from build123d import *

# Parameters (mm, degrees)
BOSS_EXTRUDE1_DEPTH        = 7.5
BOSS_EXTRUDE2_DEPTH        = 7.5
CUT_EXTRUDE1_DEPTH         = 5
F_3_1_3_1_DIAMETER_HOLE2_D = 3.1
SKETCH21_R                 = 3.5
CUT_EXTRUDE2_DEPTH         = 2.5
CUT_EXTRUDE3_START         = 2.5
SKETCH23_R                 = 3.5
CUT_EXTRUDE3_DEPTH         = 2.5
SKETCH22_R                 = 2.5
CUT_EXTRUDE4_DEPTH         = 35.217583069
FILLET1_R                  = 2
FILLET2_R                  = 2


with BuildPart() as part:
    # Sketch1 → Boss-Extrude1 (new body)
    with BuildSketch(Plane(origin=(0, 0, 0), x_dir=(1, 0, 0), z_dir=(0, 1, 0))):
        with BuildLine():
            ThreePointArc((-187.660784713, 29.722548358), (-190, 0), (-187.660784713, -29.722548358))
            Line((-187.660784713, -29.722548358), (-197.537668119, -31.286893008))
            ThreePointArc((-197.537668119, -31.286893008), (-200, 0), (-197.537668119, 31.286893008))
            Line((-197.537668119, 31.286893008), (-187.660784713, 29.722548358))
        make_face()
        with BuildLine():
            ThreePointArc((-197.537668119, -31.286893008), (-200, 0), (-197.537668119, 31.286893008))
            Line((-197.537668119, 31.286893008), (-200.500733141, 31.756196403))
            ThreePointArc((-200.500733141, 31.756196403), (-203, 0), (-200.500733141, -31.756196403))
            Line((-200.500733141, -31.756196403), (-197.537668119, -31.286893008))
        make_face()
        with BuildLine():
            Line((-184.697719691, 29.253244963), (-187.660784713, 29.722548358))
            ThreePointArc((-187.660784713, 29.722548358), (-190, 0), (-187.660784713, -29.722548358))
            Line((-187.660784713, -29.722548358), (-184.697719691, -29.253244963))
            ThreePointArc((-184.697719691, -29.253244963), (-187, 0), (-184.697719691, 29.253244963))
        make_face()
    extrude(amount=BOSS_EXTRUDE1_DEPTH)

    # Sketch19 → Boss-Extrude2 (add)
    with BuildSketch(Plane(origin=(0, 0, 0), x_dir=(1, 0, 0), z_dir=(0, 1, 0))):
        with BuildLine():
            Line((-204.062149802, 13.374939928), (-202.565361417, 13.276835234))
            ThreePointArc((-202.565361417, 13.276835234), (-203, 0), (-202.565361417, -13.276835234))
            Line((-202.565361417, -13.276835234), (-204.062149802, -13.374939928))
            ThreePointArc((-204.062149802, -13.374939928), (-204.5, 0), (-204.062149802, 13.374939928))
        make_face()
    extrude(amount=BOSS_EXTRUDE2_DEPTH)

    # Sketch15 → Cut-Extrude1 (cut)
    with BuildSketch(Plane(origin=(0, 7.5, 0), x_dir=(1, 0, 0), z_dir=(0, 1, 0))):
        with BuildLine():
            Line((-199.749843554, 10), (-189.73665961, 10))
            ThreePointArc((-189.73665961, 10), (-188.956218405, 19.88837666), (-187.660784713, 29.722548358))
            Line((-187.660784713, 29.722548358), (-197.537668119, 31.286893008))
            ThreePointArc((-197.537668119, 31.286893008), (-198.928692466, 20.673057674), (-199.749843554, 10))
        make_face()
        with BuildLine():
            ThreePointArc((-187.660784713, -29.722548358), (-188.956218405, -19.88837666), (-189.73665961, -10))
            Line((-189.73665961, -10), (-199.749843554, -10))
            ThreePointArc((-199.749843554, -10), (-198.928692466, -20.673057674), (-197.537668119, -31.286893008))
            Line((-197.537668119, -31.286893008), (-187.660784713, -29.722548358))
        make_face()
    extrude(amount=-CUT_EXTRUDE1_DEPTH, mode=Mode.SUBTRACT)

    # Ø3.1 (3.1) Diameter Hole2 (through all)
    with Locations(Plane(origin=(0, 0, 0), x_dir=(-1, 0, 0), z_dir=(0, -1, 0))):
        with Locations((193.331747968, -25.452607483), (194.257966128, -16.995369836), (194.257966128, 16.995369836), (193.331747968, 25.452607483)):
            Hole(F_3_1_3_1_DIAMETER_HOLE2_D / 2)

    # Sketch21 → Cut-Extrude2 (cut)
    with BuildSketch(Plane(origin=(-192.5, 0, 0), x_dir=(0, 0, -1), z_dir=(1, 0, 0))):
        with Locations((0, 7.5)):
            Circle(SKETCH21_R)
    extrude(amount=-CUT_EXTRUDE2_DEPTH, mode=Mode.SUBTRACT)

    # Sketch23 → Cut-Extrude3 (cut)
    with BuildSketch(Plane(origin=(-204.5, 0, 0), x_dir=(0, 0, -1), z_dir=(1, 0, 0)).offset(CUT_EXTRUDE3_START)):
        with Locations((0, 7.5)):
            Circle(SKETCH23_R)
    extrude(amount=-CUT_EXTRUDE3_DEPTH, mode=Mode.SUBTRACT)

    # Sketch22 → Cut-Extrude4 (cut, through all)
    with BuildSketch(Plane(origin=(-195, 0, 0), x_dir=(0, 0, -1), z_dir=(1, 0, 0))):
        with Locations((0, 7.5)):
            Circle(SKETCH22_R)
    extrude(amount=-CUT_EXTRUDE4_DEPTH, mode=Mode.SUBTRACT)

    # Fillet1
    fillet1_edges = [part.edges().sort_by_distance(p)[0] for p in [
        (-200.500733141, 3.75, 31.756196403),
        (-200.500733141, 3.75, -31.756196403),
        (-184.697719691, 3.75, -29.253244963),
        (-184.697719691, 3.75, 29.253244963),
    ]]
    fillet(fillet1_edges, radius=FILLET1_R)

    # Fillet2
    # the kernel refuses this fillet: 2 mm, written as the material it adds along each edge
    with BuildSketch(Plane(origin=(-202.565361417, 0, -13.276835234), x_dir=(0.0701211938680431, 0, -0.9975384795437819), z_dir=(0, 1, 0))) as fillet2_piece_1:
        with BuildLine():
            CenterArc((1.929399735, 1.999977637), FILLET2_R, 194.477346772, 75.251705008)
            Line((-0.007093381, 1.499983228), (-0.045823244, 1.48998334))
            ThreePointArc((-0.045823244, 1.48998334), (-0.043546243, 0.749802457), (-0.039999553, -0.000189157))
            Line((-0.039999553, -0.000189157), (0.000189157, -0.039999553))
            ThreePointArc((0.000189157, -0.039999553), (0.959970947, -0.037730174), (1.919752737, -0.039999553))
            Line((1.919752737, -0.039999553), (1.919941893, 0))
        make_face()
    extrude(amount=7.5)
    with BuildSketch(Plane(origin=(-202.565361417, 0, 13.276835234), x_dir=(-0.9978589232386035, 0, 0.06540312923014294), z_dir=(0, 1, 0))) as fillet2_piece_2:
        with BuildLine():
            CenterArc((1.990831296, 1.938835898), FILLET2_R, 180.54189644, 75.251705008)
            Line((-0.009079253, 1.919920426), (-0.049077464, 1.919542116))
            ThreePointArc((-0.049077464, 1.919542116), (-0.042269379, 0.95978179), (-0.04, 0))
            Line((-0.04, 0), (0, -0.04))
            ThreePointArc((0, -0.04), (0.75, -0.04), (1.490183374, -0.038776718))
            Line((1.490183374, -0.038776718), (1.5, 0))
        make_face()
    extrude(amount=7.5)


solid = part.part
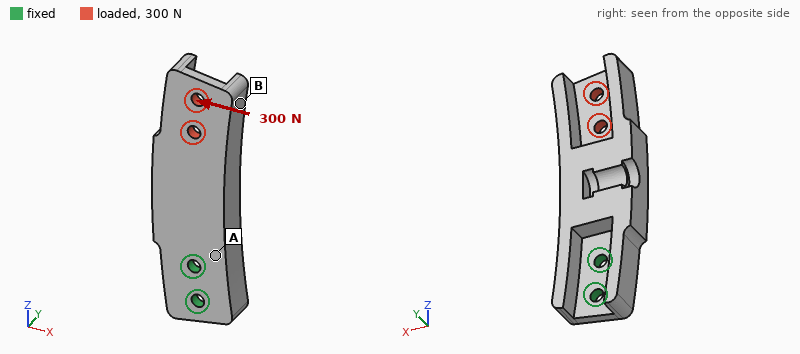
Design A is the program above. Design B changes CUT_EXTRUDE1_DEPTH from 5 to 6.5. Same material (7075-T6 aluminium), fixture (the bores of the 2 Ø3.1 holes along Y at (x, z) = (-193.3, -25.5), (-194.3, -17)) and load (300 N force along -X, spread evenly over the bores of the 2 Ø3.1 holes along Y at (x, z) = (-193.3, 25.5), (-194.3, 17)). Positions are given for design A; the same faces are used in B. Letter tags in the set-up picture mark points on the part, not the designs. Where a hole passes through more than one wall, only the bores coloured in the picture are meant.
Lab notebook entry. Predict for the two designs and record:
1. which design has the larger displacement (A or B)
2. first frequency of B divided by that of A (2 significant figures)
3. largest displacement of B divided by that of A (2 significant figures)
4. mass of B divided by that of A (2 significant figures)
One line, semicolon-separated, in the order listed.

B; 0.59; 2.0; 0.89
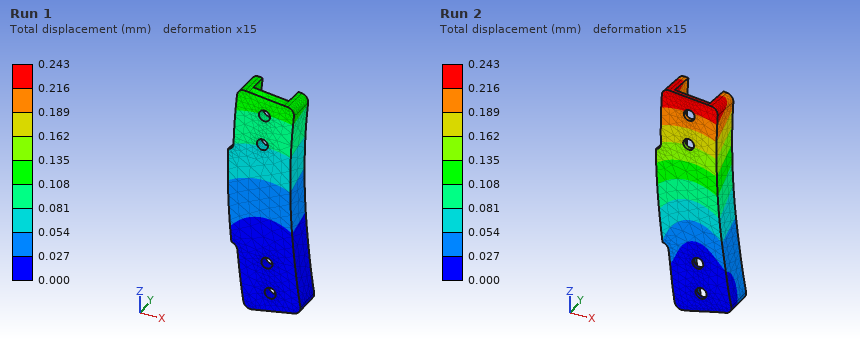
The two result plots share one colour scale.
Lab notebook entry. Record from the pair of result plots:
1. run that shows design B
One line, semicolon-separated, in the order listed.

Run 2
